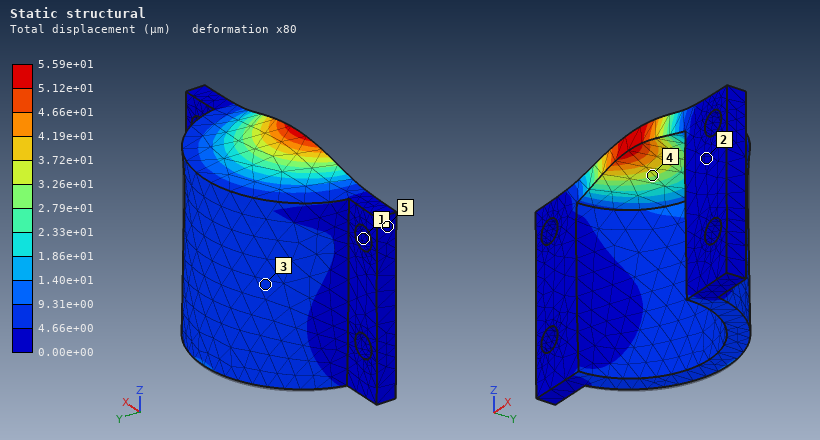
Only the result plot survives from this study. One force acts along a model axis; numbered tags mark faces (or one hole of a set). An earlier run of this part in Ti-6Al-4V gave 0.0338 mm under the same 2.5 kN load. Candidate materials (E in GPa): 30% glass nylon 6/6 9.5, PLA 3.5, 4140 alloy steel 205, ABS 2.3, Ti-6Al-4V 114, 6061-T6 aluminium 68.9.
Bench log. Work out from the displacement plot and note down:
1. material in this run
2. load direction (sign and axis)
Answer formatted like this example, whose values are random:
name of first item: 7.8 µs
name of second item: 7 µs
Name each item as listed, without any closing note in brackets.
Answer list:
material in this run: 6061-T6 aluminium
load direction: +Z
